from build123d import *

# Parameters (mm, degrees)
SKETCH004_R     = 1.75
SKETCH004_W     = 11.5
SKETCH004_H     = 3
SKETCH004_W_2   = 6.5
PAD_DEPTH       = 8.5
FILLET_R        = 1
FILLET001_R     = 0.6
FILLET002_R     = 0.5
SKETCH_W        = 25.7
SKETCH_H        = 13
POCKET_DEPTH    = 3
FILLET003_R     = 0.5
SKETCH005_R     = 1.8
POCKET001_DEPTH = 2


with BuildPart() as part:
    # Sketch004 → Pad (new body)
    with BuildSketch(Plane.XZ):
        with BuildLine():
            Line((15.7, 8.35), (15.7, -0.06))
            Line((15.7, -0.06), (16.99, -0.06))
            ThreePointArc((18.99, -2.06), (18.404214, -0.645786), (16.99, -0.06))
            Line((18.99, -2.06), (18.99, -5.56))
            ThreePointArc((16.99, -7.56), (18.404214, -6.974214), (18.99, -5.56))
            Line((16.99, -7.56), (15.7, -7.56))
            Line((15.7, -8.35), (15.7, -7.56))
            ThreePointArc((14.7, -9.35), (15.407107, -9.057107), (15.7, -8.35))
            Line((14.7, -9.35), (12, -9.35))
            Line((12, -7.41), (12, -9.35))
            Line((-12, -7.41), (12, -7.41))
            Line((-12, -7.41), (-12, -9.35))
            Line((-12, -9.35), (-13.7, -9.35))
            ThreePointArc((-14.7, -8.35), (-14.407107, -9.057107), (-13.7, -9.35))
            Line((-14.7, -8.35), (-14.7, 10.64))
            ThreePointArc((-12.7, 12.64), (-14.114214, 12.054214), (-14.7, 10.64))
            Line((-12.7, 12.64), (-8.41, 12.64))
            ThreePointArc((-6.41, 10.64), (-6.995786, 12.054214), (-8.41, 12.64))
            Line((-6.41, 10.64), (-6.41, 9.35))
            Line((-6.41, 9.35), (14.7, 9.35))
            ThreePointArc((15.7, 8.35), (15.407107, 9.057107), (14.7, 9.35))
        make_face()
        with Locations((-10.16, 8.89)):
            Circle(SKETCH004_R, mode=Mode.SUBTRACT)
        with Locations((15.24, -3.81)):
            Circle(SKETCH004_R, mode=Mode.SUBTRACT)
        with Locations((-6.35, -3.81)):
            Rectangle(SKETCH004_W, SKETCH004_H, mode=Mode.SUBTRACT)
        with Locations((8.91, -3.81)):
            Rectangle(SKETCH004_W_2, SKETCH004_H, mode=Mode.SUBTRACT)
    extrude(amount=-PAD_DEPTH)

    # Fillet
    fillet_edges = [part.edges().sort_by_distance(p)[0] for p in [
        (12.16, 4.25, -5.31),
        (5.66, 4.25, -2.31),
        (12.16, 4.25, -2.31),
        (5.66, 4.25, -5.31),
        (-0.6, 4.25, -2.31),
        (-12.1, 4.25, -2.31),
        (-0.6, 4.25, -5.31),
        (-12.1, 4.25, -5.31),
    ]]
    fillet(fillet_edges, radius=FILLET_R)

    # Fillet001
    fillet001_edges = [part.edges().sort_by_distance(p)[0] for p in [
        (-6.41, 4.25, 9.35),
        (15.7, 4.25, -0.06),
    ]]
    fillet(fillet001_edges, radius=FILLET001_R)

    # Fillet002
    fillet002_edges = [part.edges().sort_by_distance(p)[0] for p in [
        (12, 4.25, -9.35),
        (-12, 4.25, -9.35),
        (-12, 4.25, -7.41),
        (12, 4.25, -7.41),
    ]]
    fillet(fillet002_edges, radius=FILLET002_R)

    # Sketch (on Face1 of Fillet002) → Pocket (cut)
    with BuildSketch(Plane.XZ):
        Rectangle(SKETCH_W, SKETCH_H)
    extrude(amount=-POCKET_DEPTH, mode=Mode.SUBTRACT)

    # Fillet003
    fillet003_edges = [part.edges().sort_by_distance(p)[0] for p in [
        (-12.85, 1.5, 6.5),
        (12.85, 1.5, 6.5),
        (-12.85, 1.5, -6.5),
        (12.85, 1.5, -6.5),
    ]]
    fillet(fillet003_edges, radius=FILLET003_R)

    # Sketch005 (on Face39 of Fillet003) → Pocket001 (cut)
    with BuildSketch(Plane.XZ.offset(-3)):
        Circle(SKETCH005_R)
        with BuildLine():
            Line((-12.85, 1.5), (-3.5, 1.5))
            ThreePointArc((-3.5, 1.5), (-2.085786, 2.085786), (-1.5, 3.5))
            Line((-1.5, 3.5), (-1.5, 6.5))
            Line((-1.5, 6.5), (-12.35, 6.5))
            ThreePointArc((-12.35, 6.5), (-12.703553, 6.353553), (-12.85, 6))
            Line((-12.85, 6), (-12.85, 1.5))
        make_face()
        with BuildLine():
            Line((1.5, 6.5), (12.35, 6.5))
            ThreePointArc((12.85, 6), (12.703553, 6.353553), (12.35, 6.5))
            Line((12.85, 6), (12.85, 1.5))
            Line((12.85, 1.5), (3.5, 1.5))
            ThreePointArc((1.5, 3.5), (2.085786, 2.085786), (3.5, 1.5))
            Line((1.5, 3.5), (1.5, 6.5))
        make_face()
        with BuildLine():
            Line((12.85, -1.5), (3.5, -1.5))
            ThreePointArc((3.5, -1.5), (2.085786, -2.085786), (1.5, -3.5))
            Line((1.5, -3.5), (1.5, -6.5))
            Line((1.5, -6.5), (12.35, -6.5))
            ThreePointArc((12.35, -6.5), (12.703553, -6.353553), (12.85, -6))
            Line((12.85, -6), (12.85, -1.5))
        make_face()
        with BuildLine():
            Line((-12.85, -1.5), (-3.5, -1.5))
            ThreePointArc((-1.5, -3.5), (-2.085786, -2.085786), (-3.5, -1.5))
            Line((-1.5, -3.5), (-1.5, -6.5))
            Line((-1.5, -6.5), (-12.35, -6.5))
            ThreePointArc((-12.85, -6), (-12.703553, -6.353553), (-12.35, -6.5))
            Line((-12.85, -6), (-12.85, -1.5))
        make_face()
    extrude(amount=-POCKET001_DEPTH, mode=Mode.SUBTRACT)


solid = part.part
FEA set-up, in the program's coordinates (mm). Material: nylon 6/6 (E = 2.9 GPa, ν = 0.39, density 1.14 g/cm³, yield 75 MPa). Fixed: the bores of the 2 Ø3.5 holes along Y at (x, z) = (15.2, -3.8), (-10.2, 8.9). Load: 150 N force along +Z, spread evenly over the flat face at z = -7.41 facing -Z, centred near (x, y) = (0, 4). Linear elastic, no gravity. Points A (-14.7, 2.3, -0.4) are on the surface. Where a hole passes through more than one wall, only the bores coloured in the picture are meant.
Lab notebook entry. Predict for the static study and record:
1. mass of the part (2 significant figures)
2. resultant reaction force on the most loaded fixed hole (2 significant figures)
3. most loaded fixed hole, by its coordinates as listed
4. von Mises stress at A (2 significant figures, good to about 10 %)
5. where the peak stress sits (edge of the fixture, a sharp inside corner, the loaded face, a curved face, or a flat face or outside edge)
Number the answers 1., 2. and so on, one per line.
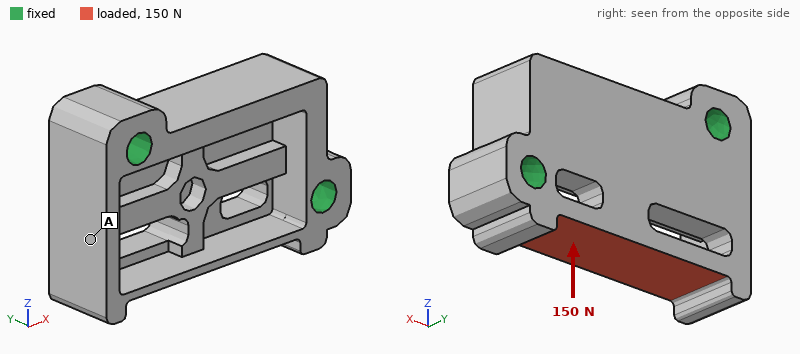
1. 3.4 g
2. 90 N
3. (-10.2, 8.9)
4. 3.8 MPa
5. the loaded face
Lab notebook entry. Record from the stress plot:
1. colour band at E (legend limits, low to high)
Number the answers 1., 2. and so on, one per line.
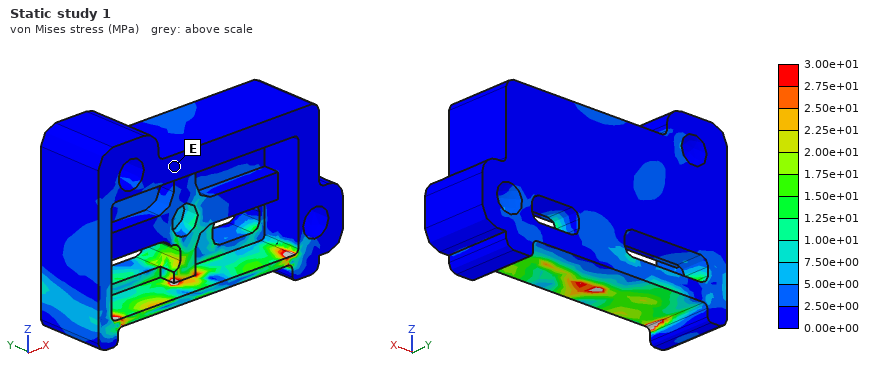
1. 0.00e+00 to 2.50e+00 MPa
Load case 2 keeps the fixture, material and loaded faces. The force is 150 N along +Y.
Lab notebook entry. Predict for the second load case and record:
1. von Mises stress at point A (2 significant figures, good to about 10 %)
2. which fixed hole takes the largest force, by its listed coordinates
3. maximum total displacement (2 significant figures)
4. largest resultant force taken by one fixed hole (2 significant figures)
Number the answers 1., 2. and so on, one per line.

1. 7.8 MPa
2. (15.2, -3.8)
3. 0.28 mm
4. 95 N
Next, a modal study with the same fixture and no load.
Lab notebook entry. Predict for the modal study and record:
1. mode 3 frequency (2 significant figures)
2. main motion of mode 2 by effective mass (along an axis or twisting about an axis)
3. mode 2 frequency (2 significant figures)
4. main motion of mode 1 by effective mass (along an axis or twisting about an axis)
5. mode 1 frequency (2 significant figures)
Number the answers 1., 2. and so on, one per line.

1. 9400 Hz
2. along Y
3. 8600 Hz
4. along Y
5. 5400 Hz
